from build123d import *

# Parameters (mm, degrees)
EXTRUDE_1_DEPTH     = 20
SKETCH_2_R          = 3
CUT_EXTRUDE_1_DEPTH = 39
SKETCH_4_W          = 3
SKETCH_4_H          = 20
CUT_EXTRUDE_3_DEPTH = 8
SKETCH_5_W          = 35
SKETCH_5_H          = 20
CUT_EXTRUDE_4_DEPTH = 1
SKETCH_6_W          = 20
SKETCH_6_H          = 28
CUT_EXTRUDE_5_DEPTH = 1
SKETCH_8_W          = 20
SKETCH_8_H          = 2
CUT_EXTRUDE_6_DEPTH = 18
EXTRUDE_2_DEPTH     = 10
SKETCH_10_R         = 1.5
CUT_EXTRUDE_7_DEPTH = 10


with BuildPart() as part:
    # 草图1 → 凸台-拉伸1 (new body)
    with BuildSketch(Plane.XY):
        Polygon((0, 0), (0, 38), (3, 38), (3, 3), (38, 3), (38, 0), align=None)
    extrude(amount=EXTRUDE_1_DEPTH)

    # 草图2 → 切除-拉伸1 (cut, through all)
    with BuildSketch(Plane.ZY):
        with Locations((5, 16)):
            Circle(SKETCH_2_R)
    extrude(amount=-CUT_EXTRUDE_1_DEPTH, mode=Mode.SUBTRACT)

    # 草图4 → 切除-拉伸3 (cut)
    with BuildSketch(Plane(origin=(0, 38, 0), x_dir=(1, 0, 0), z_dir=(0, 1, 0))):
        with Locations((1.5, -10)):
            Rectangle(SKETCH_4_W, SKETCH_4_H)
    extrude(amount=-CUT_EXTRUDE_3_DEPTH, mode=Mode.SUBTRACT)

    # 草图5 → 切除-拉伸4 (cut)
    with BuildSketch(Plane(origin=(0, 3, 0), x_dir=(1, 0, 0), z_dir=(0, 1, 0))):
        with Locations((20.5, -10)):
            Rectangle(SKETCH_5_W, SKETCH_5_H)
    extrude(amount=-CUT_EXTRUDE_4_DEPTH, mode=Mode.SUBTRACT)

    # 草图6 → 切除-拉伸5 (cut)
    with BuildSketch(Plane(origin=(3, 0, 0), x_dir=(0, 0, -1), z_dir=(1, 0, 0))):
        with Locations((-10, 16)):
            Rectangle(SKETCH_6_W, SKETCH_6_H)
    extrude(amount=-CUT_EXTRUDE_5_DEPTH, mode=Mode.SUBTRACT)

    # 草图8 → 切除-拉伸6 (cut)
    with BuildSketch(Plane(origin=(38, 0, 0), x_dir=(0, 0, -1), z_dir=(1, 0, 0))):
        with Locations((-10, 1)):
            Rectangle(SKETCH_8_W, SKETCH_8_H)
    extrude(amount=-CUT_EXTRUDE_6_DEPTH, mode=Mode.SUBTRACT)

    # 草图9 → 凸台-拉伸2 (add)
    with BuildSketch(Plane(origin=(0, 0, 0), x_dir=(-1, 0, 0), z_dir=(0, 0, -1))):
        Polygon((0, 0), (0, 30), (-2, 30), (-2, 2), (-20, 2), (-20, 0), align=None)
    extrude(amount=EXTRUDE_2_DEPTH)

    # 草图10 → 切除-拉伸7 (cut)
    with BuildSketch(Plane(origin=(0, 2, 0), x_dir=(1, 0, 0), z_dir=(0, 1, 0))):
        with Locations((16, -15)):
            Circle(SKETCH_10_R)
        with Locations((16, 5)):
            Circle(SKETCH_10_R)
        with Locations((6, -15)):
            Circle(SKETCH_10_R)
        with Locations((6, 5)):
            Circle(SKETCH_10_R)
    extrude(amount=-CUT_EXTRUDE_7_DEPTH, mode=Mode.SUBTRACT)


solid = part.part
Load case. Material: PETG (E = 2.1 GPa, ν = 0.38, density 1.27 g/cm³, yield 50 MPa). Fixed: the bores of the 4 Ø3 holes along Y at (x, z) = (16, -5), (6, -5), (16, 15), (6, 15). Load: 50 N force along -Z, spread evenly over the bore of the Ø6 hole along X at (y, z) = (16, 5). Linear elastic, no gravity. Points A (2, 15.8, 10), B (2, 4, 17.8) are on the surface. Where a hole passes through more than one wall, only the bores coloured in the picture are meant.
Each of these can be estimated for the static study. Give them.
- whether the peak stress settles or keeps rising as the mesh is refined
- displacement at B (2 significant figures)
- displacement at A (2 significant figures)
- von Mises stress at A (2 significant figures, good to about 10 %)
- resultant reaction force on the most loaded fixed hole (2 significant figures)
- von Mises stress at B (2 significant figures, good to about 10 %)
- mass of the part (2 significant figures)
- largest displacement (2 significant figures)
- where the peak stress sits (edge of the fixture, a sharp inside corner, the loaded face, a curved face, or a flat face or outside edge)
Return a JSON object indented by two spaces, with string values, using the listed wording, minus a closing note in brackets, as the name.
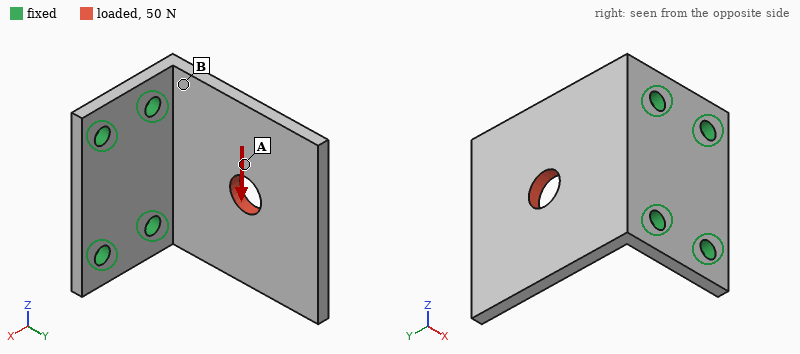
{
  "whether the peak stress settles or keeps rising as the mesh is refined": "keeps rising",
  "displacement at B": "0.074 mm",
  "displacement at A": "0.12 mm",
  "von Mises stress at A": "2.4 MPa",
  "resultant reaction force on the most loaded fixed hole": "45 N",
  "von Mises stress at B": "5.5 MPa",
  "mass of the part": "3.5 g",
  "largest displacement": "0.27 mm",
  "where the peak stress sits": "edge of the fixture"
}
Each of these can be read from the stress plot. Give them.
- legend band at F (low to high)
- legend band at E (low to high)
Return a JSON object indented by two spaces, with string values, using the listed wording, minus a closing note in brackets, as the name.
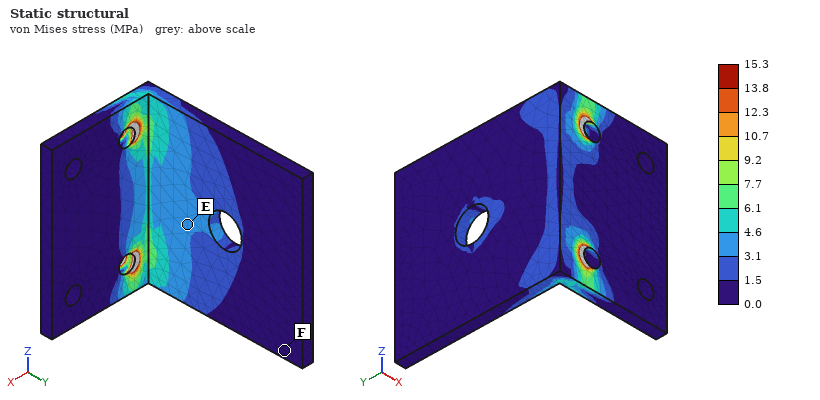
{
  "legend band at F": "0.0 to 1.5 MPa",
  "legend band at E": "3.1 to 4.6 MPa"
}
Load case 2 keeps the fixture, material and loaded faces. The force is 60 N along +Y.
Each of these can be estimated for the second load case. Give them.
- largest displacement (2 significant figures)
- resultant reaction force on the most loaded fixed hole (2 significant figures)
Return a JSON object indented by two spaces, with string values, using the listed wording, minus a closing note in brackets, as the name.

{
  "largest displacement": "0.45 mm",
  "resultant reaction force on the most loaded fixed hole": "33 N"
}
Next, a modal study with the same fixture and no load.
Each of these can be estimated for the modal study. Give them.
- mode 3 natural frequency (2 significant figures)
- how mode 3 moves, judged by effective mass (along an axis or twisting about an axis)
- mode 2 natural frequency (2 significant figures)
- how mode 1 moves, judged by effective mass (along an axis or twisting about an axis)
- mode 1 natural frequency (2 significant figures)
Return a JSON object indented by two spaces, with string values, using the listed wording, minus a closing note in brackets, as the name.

{
  "mode 3 natural frequency": "2000 Hz",
  "how mode 3 moves, judged by effective mass": "along Z",
  "mode 2 natural frequency": "1000 Hz",
  "how mode 1 moves, judged by effective mass": "along X",
  "mode 1 natural frequency": "410 Hz"
}
